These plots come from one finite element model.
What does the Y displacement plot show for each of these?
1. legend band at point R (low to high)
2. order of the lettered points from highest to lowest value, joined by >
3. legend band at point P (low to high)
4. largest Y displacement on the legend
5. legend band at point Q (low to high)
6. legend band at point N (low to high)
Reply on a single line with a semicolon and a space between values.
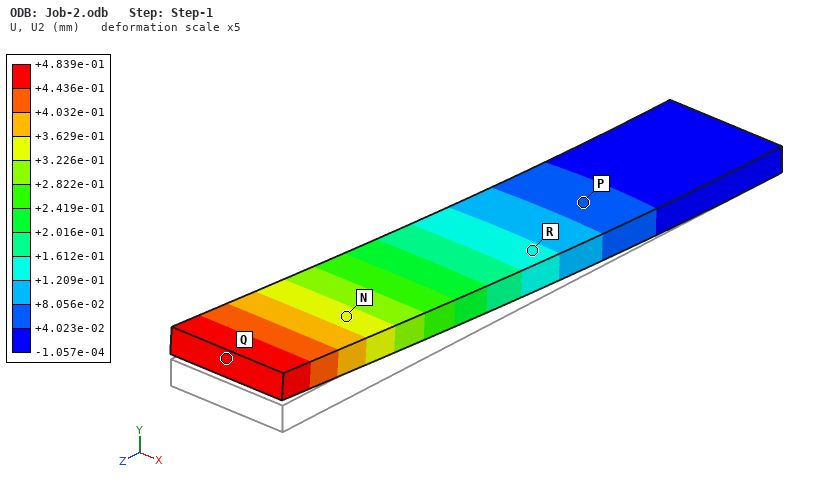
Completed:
+1.209e-01 to +1.612e-01 mm; Q > N > R > P; +4.023e-02 to +8.056e-02 mm; +4.839e-01 mm; +4.436e-01 to +4.839e-01 mm; +3.226e-01 to +3.629e-01 mm
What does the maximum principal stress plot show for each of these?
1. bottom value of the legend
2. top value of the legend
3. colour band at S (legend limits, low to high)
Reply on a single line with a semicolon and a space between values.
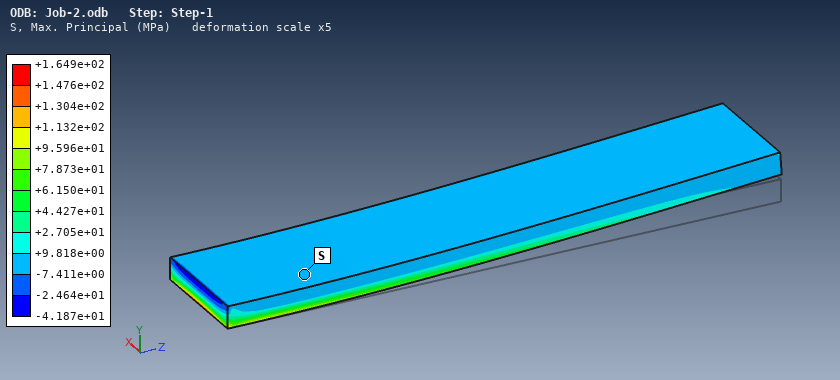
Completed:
-4.187e+01 MPa; +1.649e+02 MPa; -7.411e+00 to +9.818e+00 MPa
